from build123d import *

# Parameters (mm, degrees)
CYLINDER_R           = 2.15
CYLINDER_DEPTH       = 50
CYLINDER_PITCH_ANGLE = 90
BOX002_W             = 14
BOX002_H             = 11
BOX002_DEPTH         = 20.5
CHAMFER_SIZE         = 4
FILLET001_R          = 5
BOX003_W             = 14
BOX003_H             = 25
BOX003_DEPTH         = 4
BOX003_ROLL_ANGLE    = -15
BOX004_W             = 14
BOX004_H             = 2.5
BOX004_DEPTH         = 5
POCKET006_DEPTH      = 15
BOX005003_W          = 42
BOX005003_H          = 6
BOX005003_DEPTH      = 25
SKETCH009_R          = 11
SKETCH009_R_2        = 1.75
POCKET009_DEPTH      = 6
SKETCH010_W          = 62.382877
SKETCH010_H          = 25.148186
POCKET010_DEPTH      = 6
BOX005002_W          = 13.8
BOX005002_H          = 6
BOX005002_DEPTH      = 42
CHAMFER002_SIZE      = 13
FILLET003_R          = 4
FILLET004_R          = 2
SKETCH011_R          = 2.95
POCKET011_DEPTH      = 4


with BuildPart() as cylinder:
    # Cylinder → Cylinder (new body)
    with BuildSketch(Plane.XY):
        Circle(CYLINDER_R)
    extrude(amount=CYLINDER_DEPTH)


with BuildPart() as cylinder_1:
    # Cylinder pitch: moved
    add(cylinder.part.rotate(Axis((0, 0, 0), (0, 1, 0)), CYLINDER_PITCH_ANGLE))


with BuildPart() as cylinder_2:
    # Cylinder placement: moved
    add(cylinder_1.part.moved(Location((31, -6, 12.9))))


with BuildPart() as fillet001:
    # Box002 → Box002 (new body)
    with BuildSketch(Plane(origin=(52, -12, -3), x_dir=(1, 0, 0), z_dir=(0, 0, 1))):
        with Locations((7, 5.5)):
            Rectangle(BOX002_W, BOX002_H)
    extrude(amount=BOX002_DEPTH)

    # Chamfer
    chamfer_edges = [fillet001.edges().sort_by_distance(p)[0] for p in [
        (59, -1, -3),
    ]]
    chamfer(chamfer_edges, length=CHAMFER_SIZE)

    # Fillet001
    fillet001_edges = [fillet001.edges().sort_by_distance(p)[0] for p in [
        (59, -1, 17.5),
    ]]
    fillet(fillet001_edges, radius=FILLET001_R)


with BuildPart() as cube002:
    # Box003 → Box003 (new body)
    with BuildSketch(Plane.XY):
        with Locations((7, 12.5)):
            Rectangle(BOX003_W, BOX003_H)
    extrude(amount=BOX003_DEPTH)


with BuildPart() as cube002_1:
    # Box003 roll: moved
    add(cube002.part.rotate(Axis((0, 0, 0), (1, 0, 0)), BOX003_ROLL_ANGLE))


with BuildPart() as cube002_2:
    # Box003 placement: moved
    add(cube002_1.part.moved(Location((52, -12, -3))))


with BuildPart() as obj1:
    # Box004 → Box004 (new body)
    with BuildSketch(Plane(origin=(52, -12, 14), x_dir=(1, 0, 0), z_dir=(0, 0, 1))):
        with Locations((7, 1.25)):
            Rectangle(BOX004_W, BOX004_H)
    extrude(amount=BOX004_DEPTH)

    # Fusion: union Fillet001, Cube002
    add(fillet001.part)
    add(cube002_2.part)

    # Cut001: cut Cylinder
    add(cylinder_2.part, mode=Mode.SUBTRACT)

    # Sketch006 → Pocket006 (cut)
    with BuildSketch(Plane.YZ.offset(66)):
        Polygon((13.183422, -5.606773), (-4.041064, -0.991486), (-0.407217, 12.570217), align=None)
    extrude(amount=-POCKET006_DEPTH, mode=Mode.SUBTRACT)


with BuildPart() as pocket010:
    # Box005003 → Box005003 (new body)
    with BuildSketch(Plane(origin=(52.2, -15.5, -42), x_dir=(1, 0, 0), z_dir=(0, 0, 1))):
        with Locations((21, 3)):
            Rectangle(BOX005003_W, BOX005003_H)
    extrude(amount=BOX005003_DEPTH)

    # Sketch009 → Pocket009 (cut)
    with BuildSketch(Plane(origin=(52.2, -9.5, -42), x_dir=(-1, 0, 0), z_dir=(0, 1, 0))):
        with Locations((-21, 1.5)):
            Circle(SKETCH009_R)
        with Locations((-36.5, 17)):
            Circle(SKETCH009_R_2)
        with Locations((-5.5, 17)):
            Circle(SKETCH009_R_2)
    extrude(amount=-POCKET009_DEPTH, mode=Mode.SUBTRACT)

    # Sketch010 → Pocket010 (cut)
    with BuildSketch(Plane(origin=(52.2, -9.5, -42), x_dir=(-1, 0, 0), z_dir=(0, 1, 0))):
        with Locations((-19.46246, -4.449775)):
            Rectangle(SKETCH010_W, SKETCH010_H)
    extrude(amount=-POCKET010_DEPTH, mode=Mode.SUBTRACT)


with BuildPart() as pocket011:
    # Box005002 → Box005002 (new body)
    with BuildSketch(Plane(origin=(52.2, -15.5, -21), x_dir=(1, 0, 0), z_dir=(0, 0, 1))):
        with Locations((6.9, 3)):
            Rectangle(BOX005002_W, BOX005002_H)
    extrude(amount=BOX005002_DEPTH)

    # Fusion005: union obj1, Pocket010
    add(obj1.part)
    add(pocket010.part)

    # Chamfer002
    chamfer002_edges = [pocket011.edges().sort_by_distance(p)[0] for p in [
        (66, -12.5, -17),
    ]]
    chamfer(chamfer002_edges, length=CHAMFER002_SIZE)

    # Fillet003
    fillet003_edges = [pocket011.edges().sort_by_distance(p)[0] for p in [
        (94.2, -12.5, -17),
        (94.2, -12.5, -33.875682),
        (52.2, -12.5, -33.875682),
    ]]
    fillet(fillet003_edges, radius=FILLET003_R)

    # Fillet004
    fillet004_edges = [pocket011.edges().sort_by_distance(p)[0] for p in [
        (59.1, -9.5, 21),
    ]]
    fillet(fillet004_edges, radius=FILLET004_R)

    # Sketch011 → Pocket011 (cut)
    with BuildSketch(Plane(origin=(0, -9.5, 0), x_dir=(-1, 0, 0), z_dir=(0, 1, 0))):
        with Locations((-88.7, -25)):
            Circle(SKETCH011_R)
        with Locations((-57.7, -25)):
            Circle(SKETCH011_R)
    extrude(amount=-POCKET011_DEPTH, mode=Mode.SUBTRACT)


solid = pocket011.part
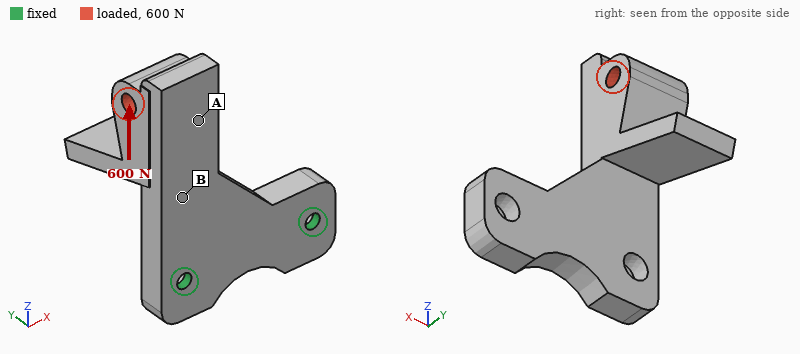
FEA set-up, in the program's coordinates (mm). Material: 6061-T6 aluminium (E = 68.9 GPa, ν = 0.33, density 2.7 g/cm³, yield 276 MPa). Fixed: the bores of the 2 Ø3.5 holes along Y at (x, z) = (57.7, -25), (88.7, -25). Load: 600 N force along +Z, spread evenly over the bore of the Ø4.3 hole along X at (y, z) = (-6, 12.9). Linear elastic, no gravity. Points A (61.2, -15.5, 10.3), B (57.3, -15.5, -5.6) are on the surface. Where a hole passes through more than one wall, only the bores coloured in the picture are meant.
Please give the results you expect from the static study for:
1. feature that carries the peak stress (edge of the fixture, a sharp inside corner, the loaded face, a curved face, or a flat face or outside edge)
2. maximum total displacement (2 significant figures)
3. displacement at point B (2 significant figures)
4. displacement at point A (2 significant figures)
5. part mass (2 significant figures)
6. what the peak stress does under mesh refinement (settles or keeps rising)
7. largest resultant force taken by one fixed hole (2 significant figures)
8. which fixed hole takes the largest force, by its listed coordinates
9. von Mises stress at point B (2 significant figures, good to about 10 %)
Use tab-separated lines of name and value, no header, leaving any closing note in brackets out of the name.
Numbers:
feature that carries the peak stress	edge of the fixture
maximum total displacement	0.28 mm
displacement at point B	0.086 mm
displacement at point A	0.20 mm
part mass	27 g
what the peak stress does under mesh refinement	keeps rising
largest resultant force taken by one fixed hole	560 N
which fixed hole takes the largest force, by its listed coordinates	(57.7, -25)
von Mises stress at point B	33 MPa
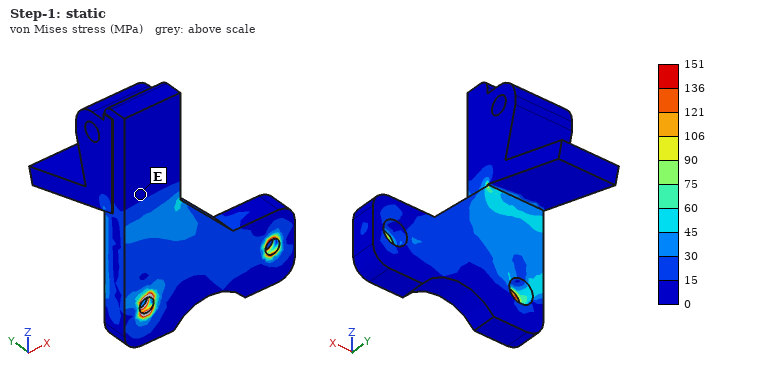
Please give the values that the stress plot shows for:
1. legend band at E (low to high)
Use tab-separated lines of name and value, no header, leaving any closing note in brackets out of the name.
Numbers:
legend band at E	0 to 15 MPa
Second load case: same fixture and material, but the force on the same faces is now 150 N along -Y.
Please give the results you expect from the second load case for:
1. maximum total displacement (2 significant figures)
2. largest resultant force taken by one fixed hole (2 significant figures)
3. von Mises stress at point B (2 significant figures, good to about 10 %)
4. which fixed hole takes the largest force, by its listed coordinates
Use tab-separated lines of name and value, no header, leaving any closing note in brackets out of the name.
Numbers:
maximum total displacement	0.29 mm
largest resultant force taken by one fixed hole	160 N
von Mises stress at point B	29 MPa
which fixed hole takes the largest force, by its listed coordinates	(57.7, -25)
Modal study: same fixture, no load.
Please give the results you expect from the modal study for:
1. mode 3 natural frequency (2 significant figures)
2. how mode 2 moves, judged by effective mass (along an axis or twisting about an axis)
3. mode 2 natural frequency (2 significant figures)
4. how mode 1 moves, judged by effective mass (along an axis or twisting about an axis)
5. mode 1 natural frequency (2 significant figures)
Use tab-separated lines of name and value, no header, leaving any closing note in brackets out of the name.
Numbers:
mode 3 natural frequency	6000 Hz
how mode 2 moves, judged by effective mass	along X
mode 2 natural frequency	4500 Hz
how mode 1 moves, judged by effective mass	along Y
mode 1 natural frequency	1300 Hz
